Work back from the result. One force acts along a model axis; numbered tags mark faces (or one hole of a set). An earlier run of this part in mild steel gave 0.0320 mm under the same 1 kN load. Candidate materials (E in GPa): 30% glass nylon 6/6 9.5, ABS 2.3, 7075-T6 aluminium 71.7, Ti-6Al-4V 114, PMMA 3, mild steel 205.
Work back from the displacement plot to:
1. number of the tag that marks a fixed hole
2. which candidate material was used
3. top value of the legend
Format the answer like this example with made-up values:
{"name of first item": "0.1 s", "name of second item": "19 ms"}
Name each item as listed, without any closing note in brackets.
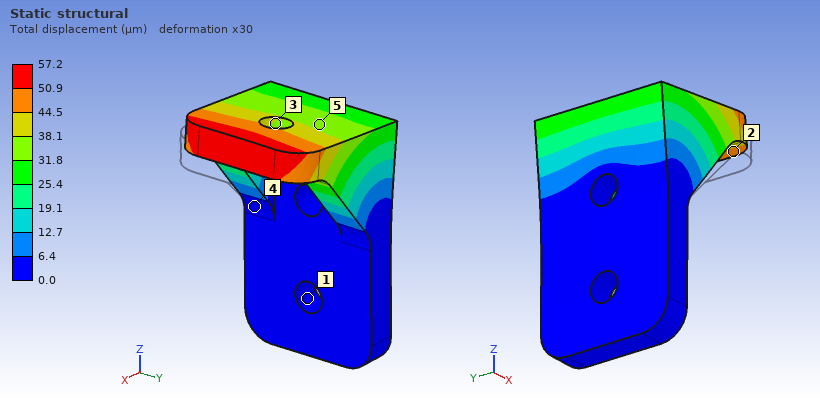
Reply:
{"number of the tag that marks a fixed hole": "1", "which candidate material was used": "Ti-6Al-4V", "top value of the legend": "57.2 µm"}
